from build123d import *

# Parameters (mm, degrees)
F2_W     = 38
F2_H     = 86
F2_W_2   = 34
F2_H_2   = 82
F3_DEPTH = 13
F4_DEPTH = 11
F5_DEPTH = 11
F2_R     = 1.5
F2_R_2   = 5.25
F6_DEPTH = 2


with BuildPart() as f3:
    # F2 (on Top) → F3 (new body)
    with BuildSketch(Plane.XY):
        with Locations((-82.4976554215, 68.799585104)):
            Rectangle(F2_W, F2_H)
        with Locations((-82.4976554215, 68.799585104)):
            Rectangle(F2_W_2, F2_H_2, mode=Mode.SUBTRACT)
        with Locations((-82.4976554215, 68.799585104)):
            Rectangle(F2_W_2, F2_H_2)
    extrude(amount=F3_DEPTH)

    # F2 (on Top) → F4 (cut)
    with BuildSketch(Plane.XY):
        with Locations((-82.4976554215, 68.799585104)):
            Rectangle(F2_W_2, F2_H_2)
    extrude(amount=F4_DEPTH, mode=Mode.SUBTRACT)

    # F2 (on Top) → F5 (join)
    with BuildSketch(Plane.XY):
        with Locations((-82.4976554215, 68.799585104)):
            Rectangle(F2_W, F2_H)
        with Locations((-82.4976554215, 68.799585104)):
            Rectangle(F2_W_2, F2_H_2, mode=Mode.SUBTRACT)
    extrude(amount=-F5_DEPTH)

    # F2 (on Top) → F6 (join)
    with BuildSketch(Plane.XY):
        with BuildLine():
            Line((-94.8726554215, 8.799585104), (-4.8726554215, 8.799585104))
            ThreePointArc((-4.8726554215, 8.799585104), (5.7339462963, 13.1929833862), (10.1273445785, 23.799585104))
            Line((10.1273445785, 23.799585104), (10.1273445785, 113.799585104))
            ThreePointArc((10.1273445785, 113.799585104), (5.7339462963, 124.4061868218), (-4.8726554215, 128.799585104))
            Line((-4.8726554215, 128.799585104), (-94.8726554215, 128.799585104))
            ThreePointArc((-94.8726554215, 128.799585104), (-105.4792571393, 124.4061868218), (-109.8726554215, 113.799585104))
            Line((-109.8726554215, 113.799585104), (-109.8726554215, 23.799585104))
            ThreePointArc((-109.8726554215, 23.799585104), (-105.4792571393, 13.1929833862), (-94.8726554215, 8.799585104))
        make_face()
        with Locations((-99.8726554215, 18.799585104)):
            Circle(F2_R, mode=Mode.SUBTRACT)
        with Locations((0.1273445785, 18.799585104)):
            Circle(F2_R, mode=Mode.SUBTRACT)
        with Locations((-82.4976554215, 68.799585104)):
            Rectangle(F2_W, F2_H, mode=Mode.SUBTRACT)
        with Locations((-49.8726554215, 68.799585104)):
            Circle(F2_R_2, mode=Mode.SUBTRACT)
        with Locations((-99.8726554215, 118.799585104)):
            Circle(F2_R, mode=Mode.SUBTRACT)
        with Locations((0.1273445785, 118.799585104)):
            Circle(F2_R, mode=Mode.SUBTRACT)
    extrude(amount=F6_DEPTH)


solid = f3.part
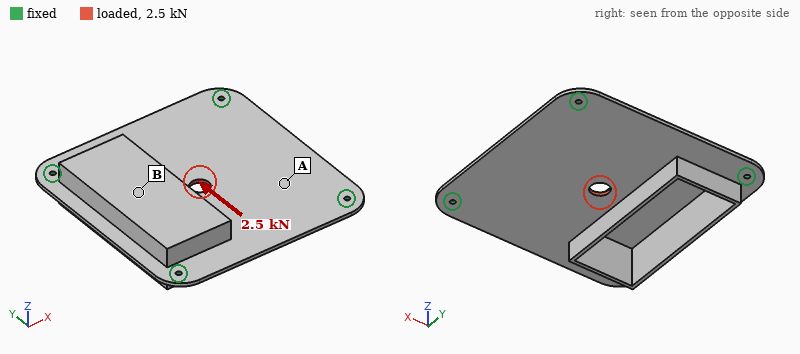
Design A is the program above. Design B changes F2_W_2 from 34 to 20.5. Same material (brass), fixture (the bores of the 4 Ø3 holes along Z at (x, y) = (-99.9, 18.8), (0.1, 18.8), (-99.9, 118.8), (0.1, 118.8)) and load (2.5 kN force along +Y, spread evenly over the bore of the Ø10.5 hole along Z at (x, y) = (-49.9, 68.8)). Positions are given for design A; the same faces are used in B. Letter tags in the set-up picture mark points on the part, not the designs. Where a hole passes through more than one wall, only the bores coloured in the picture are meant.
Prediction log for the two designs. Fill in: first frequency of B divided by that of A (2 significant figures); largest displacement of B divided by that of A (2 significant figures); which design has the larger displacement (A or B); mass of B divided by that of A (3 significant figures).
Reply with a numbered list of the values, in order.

1. 0.84
2. 0.48
3. A
4. 1.63
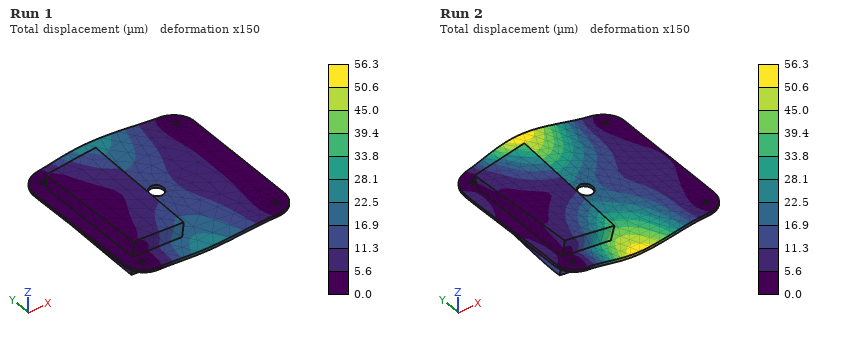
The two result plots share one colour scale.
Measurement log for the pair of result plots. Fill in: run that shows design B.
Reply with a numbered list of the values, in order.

1. Run 1
